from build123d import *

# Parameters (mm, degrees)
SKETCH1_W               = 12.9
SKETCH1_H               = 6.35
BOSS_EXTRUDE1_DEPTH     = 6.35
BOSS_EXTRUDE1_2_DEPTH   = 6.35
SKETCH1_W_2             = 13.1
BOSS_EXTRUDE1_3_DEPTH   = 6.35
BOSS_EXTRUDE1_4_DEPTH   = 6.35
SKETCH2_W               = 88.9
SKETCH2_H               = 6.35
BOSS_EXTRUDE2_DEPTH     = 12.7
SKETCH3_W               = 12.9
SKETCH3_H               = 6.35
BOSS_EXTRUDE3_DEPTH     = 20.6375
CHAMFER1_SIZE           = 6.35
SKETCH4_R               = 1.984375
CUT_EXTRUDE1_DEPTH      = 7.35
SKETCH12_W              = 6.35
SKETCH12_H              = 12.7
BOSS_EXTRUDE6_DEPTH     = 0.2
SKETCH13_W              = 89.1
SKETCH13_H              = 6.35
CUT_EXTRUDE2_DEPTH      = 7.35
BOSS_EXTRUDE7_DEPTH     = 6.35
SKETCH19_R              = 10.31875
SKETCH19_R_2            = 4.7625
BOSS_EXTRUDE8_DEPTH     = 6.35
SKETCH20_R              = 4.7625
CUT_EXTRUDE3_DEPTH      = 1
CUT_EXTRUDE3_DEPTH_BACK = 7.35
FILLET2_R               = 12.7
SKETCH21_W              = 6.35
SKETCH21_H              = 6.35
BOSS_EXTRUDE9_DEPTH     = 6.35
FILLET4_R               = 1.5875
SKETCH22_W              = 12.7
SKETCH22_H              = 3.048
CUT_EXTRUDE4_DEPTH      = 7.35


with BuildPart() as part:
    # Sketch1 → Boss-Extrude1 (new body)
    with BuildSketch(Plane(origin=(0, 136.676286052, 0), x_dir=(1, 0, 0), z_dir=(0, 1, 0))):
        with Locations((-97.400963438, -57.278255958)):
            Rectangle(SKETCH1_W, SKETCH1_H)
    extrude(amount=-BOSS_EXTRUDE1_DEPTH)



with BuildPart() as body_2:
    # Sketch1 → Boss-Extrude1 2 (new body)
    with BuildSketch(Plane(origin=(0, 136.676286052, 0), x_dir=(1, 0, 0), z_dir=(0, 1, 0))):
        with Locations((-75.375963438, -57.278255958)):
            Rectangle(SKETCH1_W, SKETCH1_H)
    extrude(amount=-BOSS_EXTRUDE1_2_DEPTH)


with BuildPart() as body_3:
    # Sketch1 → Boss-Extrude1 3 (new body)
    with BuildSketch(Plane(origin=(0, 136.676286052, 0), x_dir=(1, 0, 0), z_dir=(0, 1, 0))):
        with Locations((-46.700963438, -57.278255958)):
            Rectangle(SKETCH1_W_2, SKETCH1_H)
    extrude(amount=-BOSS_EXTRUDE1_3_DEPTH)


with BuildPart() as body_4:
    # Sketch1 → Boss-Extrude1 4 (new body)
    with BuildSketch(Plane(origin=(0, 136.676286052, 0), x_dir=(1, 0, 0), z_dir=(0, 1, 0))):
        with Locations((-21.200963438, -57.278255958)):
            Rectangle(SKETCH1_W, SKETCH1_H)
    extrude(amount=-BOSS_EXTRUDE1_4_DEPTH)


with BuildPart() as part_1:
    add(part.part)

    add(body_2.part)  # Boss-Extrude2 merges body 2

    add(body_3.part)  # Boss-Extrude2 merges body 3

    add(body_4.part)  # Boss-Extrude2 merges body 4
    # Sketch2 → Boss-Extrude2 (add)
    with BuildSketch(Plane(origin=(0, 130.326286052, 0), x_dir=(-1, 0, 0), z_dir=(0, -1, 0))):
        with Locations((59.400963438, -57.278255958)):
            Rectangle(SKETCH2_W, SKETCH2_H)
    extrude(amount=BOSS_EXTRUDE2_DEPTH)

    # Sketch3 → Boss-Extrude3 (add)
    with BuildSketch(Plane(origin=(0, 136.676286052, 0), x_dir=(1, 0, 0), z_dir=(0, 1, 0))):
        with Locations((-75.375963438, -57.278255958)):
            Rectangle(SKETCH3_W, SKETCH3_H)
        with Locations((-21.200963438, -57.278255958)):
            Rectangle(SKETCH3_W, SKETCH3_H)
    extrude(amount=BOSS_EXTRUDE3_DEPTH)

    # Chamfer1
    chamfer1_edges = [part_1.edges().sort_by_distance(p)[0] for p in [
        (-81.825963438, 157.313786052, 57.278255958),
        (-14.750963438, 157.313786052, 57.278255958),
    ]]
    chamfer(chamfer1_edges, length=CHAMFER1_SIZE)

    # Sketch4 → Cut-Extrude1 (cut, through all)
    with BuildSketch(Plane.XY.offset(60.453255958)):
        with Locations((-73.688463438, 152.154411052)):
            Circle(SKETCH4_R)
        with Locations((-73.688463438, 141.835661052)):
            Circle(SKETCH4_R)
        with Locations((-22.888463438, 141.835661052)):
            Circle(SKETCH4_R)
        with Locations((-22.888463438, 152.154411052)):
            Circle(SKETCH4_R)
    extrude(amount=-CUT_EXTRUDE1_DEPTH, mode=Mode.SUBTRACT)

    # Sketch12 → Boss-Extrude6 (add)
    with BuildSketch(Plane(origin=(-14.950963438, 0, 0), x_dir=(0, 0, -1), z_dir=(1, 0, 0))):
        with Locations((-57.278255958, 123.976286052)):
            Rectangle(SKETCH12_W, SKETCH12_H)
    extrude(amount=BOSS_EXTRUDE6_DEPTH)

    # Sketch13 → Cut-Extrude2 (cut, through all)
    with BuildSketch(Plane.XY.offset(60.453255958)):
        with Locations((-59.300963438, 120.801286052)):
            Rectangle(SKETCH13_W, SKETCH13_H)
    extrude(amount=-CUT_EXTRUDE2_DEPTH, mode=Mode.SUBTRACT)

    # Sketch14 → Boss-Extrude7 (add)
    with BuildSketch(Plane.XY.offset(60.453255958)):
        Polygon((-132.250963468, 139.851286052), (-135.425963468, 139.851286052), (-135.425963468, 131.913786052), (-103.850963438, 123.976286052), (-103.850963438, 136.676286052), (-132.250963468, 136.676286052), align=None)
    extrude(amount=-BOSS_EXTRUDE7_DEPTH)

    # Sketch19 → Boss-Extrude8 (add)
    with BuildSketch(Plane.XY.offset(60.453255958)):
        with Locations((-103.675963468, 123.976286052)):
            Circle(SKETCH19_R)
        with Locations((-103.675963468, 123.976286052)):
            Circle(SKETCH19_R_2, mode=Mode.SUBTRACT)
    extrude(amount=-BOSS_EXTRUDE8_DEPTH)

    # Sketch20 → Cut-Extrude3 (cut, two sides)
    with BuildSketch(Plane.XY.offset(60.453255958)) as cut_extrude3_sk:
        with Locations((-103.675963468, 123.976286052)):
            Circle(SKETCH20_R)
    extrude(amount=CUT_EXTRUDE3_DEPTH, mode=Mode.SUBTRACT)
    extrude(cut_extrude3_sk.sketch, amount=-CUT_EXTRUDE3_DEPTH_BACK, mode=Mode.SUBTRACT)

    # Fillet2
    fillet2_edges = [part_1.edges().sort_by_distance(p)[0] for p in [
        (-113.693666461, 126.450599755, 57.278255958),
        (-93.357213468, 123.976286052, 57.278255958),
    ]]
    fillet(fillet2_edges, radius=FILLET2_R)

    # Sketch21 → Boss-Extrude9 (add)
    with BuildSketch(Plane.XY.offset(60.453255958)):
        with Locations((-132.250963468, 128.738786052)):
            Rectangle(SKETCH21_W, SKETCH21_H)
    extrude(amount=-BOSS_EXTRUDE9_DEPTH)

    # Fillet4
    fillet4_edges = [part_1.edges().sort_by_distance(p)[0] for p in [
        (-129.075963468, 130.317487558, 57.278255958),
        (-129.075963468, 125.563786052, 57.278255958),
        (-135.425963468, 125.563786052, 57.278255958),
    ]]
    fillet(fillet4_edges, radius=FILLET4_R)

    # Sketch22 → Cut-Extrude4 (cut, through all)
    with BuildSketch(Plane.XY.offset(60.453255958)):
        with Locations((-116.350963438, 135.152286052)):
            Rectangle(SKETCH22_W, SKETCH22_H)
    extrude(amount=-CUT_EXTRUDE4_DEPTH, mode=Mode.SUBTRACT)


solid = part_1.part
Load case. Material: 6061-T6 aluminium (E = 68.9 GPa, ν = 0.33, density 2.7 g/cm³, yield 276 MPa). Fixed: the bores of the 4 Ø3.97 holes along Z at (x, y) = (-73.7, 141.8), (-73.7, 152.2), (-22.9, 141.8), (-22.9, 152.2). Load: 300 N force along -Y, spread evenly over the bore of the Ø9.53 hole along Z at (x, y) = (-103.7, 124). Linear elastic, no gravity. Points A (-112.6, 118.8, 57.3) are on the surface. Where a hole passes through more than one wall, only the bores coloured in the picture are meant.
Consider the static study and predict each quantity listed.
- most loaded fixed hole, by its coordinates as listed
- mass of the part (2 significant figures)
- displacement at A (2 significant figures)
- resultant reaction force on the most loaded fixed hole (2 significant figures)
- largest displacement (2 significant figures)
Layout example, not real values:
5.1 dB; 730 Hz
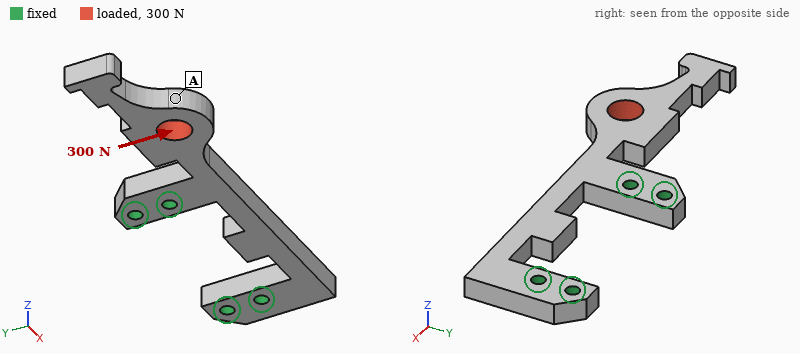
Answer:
(-22.9, 141.8); 30 g; 0.27 mm; 370 N; 0.47 mm
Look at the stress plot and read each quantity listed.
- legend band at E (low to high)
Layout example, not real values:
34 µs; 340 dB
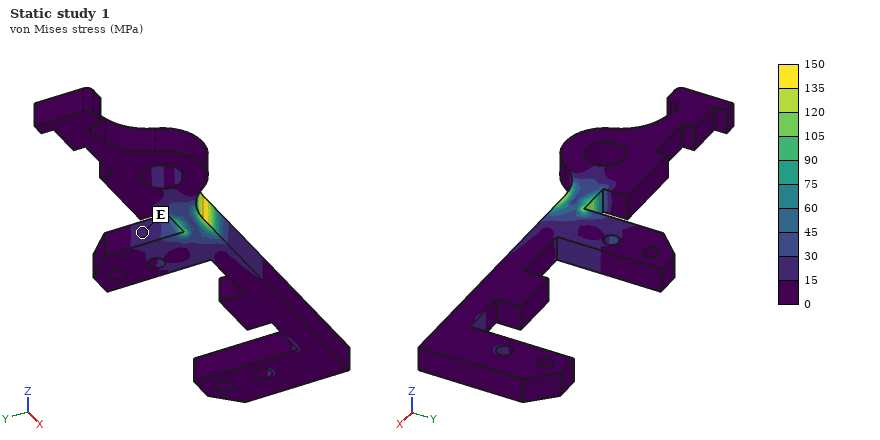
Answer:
15 to 30 MPa
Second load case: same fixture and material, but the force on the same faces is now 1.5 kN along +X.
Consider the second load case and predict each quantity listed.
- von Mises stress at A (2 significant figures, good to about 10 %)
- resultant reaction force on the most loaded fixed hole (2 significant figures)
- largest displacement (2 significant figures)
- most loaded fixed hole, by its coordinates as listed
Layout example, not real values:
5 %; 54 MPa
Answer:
15 MPa; 1.5 kN; 0.49 mm; (-73.7, 141.8)
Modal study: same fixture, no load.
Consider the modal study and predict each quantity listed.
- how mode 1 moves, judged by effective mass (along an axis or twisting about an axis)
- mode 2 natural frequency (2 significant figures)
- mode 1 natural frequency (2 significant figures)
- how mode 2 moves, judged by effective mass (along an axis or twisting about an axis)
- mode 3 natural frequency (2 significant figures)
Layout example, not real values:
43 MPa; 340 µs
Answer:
along Z; 1400 Hz; 1100 Hz; along Y; 4100 Hz
